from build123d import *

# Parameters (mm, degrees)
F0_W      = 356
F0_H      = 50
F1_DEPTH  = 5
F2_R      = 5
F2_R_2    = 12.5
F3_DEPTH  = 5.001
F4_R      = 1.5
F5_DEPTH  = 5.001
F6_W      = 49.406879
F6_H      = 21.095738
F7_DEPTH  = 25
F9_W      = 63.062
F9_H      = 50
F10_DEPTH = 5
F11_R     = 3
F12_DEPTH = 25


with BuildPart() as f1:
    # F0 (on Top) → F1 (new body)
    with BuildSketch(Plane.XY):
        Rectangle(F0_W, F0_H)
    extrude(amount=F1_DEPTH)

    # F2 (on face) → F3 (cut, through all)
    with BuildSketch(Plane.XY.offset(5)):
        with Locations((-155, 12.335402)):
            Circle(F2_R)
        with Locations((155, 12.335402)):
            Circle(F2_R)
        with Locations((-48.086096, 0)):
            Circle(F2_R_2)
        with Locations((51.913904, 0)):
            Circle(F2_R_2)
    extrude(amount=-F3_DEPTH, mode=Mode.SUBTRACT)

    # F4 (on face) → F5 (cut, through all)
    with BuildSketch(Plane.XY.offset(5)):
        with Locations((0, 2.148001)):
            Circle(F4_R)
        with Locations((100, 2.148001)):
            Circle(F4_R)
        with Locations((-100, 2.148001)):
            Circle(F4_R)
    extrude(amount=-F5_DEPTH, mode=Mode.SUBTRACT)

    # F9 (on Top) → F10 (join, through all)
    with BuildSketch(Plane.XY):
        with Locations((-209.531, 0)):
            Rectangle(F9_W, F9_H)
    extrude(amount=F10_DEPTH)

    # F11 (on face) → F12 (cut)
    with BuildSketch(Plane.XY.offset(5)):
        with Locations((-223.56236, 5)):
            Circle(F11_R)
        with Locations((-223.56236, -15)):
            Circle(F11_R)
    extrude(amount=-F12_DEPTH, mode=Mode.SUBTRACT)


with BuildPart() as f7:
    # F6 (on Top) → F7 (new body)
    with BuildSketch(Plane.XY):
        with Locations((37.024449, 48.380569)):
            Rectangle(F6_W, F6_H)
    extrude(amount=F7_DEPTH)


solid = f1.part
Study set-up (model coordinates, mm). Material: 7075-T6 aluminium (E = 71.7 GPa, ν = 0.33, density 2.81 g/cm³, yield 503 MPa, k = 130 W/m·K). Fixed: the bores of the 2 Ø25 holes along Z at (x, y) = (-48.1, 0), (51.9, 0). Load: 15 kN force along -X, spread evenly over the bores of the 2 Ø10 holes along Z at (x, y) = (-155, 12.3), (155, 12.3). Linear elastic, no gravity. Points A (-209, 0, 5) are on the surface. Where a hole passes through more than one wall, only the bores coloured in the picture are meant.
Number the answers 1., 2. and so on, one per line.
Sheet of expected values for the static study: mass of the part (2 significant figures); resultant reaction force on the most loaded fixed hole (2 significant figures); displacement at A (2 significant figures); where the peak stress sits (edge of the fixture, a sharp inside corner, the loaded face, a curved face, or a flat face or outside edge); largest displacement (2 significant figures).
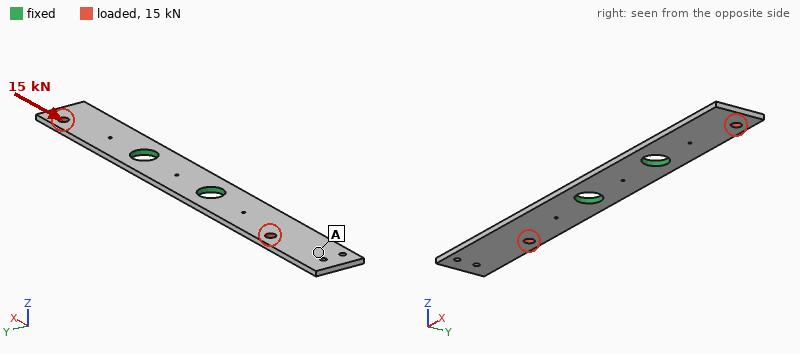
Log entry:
1. 280 g
2. 7.5 kN
3. 0.30 mm
4. the loaded face
5. 0.41 mm
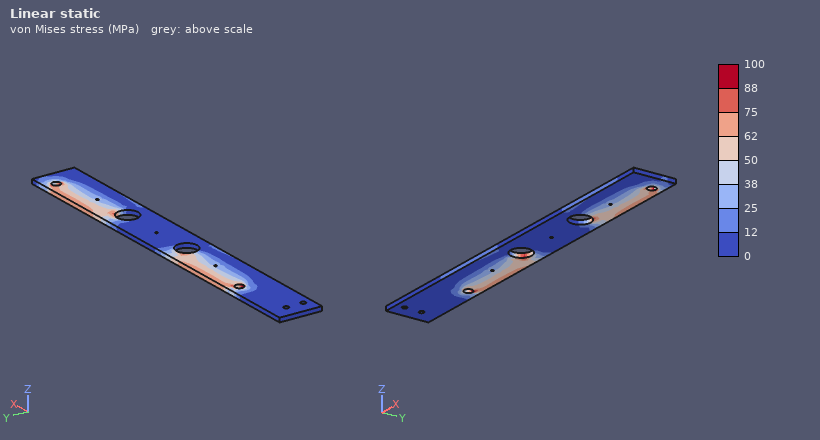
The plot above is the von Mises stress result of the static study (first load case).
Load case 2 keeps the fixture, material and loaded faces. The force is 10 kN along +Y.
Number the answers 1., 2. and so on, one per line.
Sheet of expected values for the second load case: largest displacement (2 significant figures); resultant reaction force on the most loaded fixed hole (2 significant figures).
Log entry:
1. 1.4 mm
2. 5.0 kN
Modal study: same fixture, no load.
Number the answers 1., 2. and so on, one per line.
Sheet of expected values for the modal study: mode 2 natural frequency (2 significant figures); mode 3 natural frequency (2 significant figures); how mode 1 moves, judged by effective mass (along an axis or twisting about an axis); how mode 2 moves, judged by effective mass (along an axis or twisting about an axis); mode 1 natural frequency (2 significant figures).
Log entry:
1. 310 Hz
2. 770 Hz
3. along Z
4. along Z
5. 120 Hz
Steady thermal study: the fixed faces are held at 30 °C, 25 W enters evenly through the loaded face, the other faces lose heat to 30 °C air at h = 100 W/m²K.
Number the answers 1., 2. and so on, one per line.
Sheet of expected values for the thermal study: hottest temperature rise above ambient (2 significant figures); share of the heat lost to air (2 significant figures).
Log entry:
1. 18 K
2. 80 %
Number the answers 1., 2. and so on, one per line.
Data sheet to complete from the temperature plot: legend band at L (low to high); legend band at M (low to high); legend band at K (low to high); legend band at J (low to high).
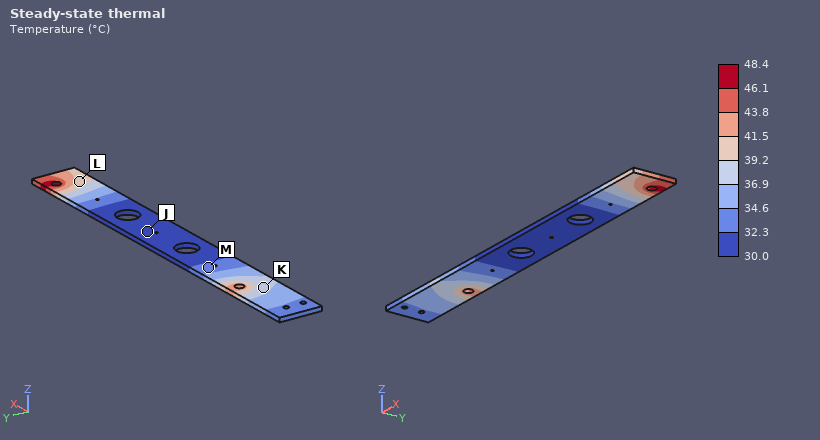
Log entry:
1. 39.2 to 41.5 °C
2. 32.3 to 34.6 °C
3. 36.9 to 39.2 °C
4. 30.0 to 32.3 °C
